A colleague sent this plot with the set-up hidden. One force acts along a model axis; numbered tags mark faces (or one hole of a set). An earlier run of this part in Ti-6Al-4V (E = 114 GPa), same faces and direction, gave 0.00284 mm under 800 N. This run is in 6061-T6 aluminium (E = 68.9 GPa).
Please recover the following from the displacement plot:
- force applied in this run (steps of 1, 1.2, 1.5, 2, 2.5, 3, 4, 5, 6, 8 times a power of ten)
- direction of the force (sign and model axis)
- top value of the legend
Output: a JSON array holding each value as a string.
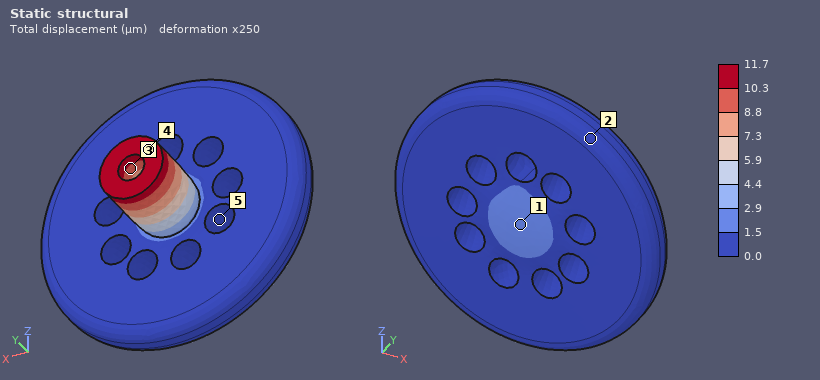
["2 kN", "-Y", "11.7 µm"]
